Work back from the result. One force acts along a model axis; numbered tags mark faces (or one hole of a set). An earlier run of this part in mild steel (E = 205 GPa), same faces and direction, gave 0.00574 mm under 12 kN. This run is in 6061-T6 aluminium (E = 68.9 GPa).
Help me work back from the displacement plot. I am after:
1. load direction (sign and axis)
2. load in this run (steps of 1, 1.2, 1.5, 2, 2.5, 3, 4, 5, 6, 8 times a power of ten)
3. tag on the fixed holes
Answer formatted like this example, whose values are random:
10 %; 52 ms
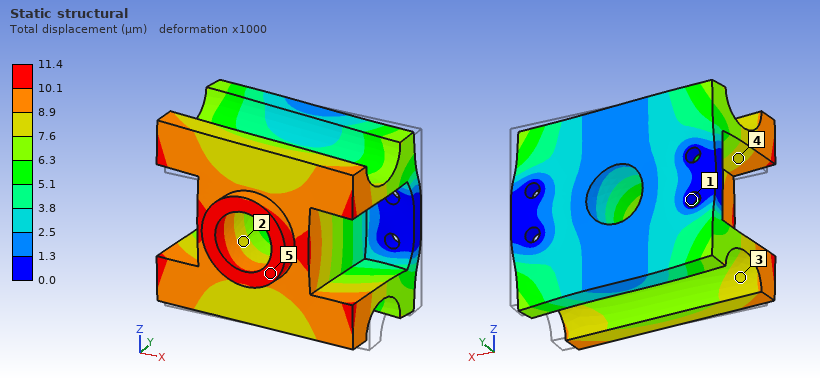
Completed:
-X; 8 kN; 1
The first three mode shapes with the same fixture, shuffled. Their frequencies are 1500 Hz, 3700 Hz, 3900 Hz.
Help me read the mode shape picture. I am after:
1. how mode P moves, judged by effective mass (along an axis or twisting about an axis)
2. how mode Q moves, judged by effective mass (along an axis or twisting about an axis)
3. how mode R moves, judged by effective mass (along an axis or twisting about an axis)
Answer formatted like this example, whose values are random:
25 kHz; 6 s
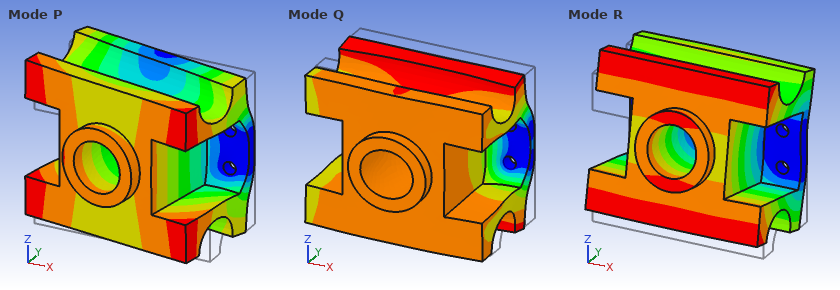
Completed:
along X; along Y; along Z
